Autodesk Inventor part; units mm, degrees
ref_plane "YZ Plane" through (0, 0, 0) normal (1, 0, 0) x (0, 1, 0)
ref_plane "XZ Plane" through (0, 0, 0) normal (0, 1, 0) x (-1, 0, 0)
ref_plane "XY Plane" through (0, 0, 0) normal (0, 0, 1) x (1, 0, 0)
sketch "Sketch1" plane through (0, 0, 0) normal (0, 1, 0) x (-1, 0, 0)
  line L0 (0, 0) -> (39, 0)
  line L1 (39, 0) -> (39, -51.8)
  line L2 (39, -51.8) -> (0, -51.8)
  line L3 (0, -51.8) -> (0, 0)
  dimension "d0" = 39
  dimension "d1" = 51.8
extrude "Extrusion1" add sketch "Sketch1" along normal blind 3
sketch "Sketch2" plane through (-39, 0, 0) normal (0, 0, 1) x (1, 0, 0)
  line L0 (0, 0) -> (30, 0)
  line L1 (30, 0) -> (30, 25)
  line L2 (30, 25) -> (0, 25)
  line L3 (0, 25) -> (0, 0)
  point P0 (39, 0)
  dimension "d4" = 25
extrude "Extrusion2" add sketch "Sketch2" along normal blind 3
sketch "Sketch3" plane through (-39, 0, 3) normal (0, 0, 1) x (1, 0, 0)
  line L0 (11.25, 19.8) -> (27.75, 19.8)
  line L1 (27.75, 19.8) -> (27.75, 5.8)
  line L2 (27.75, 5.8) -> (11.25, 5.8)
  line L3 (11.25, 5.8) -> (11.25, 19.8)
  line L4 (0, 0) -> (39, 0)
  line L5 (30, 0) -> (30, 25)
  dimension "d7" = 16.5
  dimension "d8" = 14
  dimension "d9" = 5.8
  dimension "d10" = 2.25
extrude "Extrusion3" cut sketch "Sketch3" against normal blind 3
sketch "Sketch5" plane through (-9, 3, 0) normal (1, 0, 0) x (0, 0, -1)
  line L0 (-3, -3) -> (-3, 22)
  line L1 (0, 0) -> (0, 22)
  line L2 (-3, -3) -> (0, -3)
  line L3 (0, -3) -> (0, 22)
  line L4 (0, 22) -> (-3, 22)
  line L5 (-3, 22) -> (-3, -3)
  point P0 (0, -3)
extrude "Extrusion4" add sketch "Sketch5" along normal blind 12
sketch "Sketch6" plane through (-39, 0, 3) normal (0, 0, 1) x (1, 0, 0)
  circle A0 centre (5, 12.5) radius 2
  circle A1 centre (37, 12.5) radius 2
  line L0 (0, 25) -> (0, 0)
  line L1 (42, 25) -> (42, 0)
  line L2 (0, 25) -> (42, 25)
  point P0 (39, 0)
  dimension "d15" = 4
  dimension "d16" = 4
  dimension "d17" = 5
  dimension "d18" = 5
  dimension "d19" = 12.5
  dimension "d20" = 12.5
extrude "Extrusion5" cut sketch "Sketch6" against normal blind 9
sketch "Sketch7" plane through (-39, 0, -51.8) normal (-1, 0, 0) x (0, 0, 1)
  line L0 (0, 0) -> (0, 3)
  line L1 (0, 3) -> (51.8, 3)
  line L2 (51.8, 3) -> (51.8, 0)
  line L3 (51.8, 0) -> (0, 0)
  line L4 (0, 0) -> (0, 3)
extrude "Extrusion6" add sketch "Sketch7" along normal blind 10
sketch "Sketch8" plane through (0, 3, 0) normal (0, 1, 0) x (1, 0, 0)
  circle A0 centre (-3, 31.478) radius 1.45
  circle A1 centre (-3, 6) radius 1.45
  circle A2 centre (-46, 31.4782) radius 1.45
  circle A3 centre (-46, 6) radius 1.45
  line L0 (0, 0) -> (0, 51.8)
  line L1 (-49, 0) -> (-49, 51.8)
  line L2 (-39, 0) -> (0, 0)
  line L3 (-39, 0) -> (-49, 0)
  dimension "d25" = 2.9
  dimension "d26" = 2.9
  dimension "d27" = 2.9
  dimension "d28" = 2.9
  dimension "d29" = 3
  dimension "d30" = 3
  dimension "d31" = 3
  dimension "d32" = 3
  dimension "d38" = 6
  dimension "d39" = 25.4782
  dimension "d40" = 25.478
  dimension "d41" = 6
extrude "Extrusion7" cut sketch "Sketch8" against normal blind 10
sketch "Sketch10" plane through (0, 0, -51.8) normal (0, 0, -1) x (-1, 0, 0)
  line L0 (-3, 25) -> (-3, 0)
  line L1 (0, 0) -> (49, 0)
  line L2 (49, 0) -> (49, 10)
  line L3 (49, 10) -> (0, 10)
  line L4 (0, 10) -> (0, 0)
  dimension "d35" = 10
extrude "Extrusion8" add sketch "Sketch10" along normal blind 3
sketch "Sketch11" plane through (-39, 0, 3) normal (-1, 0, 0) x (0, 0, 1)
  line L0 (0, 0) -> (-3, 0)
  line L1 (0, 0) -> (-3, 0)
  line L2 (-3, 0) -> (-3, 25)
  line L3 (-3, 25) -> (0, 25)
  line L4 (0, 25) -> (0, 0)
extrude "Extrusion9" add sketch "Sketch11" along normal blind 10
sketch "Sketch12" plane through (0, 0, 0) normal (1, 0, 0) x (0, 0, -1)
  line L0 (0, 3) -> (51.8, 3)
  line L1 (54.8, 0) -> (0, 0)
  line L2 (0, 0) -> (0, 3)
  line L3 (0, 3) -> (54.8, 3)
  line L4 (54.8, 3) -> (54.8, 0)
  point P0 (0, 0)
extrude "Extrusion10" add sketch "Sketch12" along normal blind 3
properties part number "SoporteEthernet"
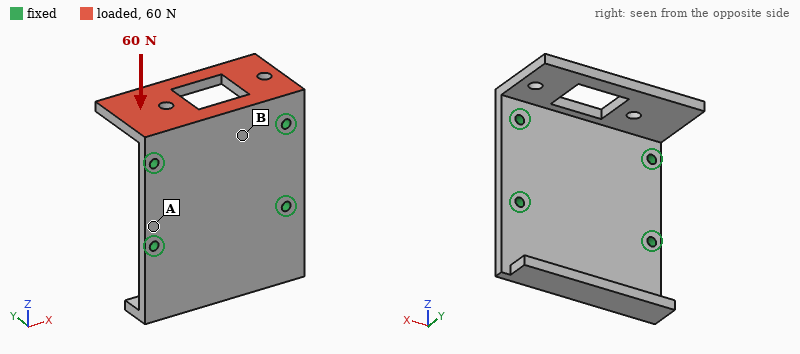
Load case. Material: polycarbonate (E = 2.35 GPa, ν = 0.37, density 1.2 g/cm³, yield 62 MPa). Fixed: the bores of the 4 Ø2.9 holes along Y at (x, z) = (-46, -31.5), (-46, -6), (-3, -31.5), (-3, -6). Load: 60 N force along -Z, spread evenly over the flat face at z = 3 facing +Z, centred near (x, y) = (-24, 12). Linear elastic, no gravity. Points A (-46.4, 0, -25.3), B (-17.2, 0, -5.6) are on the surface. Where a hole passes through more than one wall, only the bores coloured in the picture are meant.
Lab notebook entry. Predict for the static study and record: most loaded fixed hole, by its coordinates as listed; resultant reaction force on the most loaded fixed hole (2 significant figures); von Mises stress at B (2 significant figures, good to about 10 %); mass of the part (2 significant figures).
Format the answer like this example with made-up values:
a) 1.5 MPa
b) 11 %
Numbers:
a) (-3, -6)
b) 22 N
c) 3.7 MPa
d) 15 g
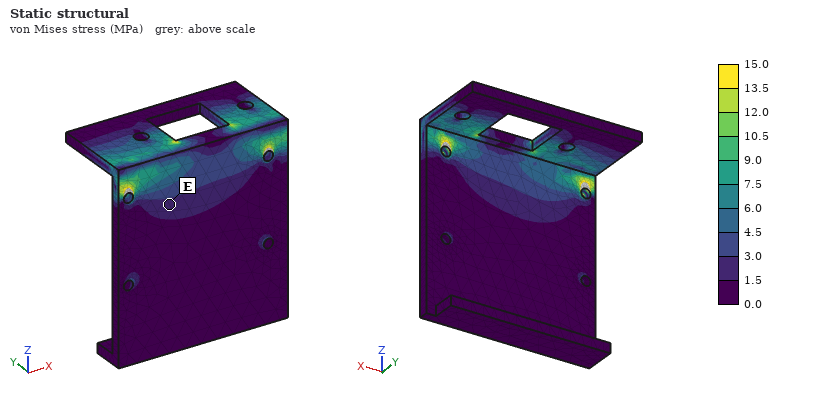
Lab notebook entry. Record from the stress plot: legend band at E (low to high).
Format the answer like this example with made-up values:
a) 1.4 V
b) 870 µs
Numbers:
a) 1.5 to 3.0 MPa
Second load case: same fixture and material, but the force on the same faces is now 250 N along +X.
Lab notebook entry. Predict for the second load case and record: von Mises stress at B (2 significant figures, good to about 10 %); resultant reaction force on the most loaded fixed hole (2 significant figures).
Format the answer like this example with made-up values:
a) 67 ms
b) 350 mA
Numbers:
a) 3.2 MPa
b) 140 N
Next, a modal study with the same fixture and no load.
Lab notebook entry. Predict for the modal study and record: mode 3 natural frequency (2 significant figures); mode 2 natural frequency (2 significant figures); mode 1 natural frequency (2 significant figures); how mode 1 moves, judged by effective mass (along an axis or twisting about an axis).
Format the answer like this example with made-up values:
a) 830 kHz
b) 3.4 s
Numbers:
a) 1200 Hz
b) 780 Hz
c) 740 Hz
d) along Y
